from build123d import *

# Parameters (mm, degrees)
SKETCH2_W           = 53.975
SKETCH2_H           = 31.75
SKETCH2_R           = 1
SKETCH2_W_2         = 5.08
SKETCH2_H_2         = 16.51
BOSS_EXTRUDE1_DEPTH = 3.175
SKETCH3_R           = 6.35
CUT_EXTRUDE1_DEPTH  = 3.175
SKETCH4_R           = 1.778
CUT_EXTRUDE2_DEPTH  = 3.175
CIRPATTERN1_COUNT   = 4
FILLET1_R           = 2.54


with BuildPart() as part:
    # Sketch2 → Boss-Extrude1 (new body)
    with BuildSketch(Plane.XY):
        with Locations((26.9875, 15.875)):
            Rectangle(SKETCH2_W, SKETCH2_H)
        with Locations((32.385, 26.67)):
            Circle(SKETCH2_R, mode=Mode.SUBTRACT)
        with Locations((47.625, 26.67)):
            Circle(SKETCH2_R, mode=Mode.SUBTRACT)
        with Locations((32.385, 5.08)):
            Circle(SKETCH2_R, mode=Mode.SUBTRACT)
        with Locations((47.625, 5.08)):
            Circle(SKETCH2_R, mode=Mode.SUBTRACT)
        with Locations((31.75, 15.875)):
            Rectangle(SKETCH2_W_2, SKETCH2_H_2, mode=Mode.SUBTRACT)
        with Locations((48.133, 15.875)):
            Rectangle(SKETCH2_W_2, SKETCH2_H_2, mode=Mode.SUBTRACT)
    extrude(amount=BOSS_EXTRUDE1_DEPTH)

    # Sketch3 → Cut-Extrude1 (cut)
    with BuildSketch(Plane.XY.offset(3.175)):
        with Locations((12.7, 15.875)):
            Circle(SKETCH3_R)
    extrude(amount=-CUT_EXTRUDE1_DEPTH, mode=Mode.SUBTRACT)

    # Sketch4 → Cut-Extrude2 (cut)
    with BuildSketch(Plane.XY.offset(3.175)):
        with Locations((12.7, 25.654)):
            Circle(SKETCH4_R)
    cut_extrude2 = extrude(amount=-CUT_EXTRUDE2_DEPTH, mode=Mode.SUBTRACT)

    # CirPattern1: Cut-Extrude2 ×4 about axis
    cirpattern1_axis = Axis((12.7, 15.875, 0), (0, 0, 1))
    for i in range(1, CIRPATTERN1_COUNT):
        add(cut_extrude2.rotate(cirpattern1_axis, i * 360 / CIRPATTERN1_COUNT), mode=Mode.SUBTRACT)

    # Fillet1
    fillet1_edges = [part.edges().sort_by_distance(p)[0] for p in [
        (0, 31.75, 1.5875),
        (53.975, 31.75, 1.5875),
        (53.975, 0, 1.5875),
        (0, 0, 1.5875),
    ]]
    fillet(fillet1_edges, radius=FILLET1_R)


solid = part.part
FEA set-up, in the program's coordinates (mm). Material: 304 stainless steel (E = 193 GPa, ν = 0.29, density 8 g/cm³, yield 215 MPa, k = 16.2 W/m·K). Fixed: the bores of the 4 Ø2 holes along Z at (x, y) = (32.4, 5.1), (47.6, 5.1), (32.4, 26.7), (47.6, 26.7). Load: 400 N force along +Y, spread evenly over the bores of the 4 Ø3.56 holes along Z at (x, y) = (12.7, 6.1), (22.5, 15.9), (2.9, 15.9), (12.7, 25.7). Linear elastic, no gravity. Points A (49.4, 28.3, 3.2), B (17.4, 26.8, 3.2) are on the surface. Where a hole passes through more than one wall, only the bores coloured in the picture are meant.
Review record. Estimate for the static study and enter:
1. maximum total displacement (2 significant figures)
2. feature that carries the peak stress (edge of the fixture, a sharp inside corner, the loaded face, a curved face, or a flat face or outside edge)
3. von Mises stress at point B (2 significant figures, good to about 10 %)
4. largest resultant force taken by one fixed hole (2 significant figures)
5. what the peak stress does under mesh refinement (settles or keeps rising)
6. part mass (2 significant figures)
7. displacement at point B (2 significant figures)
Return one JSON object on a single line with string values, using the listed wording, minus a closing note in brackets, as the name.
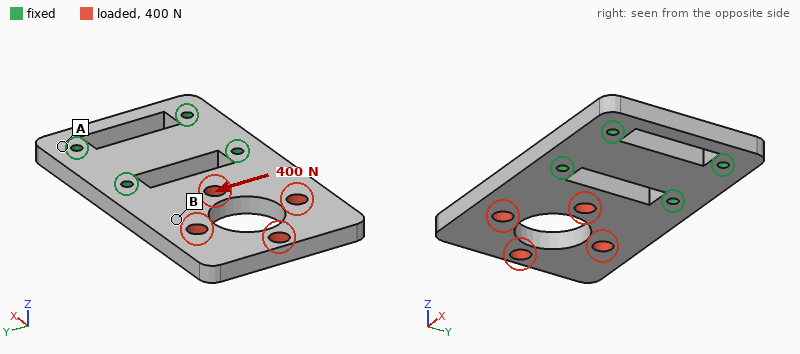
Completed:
{"maximum total displacement": "6.7 µm", "feature that carries the peak stress": "edge of the fixture", "von Mises stress at point B": "8.8 MPa", "largest resultant force taken by one fixed hole": "330 N", "what the peak stress does under mesh refinement": "keeps rising", "part mass": "35 g", "displacement at point B": "3.1 µm"}
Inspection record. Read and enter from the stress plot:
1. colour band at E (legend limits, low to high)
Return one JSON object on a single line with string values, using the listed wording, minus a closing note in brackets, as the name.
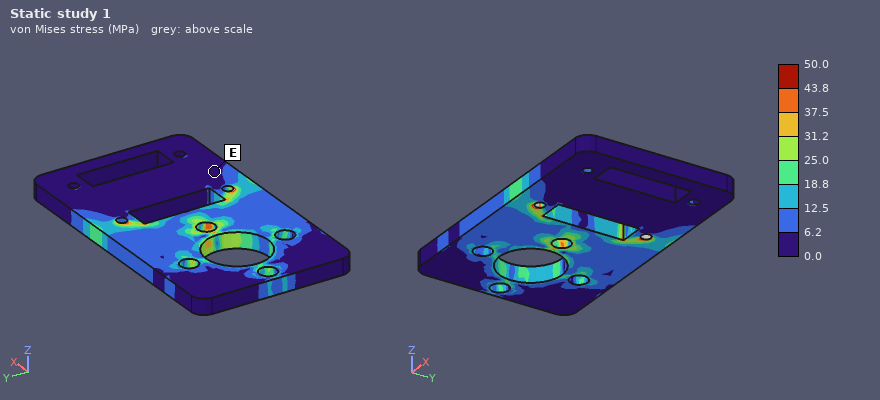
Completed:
{"colour band at E": "0.0 to 6.2 MPa"}
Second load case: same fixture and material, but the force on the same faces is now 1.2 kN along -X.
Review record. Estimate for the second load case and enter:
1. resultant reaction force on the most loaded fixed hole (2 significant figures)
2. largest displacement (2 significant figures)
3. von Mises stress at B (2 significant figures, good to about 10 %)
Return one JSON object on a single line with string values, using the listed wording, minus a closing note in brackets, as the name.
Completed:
{"resultant reaction force on the most loaded fixed hole": "560 N", "largest displacement": "4.0 µm", "von Mises stress at B": "15 MPa"}
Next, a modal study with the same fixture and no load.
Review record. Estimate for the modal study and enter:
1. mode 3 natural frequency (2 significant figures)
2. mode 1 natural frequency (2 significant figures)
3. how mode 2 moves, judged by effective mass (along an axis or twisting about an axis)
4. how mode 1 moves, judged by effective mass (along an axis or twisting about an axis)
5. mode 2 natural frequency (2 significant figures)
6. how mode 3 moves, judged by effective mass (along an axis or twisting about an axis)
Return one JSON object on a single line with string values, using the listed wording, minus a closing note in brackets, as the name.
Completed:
{"mode 3 natural frequency": "11 kHz", "mode 1 natural frequency": "2000 Hz", "how mode 2 moves, judged by effective mass": "twisting about X", "how mode 1 moves, judged by effective mass": "along Z", "mode 2 natural frequency": "5000 Hz", "how mode 3 moves, judged by effective mass": "along Y"}
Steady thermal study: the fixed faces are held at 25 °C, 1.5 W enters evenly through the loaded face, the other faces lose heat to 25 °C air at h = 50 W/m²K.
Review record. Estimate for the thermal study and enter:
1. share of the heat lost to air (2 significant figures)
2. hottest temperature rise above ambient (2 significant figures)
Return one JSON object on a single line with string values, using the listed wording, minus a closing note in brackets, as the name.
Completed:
{"share of the heat lost to air": "61 %", "hottest temperature rise above ambient": "15 K"}
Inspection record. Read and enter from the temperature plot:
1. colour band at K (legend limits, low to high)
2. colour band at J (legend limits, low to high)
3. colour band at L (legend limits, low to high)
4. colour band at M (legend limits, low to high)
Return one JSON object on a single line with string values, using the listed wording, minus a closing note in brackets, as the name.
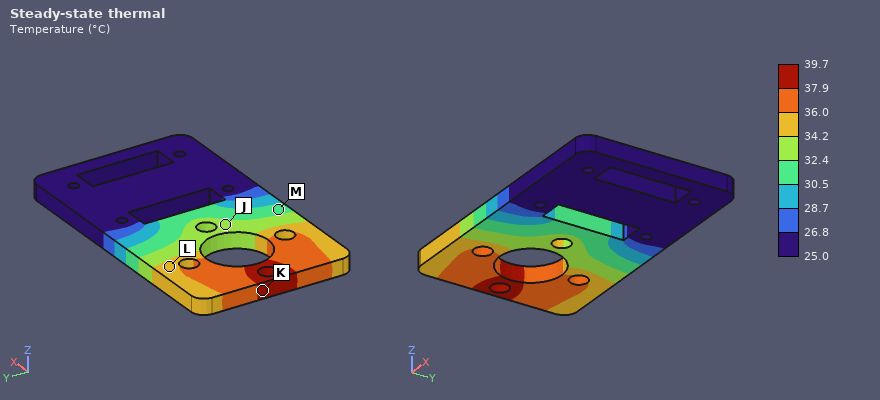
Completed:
{"colour band at K": "37.9 to 39.7 °C", "colour band at J": "32.4 to 34.2 °C", "colour band at L": "34.2 to 36.0 °C", "colour band at M": "30.5 to 32.4 °C"}
